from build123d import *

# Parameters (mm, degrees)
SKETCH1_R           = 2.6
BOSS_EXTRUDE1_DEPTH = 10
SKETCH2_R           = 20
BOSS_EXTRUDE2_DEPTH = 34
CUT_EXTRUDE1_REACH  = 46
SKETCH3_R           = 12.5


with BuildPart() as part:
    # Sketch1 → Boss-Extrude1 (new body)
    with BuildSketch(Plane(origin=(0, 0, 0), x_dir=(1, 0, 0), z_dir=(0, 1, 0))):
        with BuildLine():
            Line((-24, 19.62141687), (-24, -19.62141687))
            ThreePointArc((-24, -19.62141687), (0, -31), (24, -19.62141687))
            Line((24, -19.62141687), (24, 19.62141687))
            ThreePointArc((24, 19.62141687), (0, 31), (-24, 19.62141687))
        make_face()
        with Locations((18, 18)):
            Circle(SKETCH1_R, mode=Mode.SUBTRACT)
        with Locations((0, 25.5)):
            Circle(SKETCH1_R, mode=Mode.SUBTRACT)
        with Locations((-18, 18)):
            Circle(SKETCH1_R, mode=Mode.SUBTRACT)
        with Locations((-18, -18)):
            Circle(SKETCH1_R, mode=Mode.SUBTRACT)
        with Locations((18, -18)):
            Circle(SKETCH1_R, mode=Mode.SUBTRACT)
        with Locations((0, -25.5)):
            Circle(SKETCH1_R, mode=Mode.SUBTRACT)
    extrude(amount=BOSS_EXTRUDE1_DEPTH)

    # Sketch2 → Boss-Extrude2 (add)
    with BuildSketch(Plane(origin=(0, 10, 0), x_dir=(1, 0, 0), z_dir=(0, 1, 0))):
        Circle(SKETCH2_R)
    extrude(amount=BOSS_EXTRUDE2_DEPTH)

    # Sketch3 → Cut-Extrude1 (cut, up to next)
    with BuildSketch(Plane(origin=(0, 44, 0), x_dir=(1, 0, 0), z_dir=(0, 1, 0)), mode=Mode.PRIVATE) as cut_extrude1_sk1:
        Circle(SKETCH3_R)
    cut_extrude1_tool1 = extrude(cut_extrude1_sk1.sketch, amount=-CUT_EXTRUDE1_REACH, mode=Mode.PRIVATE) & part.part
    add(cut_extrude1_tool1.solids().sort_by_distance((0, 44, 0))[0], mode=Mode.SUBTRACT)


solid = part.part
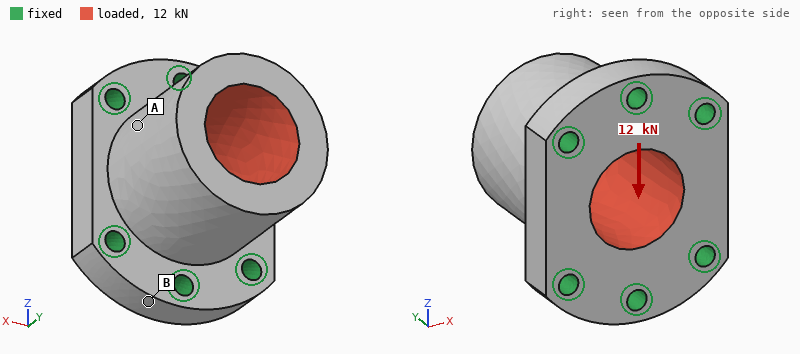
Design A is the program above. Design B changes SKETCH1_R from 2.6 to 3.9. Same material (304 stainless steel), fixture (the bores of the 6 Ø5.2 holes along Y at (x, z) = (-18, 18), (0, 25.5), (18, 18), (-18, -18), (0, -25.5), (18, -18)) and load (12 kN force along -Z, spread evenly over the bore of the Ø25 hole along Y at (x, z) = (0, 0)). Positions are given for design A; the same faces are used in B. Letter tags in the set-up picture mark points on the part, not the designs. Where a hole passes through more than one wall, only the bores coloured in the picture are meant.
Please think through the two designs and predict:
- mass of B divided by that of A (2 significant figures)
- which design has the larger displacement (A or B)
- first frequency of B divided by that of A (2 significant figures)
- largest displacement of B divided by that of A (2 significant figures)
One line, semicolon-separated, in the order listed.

0.97; A; 1.1; 0.90
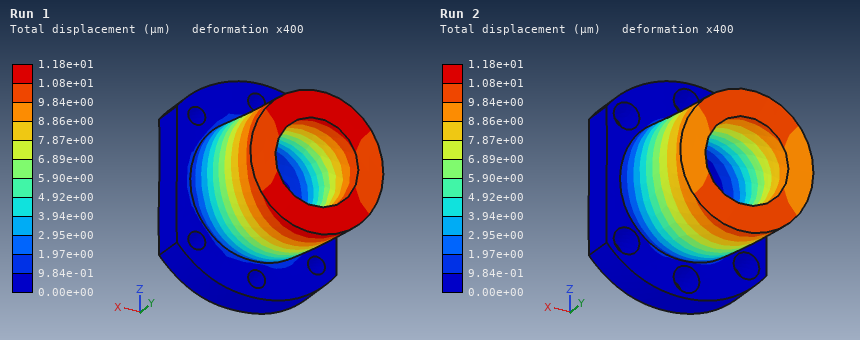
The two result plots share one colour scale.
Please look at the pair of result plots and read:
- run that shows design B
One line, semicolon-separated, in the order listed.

Run 2
